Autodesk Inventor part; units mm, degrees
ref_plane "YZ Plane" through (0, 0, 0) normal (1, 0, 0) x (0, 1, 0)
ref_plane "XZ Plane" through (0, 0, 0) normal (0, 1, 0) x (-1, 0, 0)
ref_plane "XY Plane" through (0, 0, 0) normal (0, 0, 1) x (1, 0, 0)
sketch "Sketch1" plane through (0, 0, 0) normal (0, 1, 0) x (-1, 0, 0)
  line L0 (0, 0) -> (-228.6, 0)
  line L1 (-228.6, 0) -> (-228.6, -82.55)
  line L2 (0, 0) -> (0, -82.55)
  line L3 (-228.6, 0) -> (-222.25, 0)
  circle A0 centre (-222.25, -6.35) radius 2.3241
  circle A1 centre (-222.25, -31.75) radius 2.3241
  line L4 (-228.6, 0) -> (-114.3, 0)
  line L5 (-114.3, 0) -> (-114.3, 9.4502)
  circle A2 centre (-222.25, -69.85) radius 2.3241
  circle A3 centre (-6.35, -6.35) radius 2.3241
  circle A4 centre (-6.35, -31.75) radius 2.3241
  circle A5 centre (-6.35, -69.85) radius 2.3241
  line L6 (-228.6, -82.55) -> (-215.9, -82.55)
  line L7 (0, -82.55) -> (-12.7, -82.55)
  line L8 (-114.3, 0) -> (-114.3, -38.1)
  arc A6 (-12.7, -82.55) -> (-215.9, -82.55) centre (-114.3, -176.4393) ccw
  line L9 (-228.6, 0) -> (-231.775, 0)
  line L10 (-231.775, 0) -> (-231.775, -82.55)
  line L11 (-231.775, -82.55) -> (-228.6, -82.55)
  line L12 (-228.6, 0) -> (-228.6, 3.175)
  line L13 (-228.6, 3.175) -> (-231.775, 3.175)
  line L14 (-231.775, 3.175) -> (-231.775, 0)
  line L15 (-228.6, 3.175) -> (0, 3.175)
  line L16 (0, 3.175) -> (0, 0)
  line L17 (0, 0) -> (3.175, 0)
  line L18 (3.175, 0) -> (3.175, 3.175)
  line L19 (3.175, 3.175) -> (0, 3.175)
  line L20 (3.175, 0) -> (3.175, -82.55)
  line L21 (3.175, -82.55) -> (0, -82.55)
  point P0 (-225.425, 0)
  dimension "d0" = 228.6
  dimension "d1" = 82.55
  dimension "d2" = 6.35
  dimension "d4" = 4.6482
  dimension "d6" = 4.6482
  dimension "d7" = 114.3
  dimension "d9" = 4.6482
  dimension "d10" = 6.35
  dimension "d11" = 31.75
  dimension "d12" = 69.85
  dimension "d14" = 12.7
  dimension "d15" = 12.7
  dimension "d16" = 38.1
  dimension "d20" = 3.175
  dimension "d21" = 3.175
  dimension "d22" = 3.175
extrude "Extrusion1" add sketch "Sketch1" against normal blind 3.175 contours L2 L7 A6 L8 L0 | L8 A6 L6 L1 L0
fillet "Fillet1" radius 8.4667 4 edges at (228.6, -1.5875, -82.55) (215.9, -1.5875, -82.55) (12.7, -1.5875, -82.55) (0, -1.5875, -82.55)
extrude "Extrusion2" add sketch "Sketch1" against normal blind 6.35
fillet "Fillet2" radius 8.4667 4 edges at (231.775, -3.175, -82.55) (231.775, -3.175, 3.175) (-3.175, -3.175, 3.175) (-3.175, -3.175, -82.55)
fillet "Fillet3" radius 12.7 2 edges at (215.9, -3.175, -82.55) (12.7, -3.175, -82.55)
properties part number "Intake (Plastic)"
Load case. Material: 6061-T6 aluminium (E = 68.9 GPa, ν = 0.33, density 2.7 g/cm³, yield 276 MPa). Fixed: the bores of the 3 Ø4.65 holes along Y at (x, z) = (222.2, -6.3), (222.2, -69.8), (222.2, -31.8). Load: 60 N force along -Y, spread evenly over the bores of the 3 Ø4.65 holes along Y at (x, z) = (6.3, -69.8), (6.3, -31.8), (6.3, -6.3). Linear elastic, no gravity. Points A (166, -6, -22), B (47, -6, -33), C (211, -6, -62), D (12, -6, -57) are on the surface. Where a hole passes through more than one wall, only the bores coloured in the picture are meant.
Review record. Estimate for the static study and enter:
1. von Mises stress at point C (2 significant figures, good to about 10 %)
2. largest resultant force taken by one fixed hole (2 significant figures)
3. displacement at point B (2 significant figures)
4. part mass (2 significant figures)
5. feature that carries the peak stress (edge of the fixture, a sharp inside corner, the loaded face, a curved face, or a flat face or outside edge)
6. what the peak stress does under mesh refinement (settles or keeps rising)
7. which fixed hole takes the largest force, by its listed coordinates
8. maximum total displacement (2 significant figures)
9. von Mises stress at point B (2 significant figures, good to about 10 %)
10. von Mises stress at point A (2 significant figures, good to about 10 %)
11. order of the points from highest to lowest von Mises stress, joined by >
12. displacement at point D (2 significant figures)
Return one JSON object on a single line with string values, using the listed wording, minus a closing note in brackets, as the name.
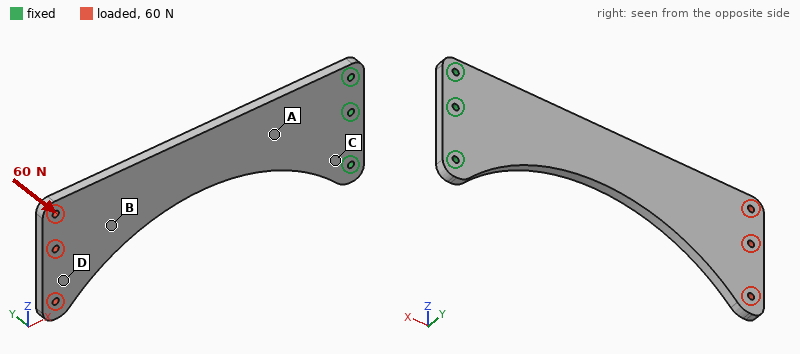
{"von Mises stress at point C": "18 MPa", "largest resultant force taken by one fixed hole": "110 N", "displacement at point B": "1.8 mm", "part mass": "240 g", "feature that carries the peak stress": "edge of the fixture", "what the peak stress does under mesh refinement": "keeps rising", "which fixed hole takes the largest force, by its listed coordinates": "(222.2, -31.8)", "maximum total displacement": "2.8 mm", "von Mises stress at point B": "6.4 MPa", "von Mises stress at point A": "27 MPa", "order of the points from highest to lowest von Mises stress, joined by >": "A > C > B > D", "displacement at point D": "2.5 mm"}
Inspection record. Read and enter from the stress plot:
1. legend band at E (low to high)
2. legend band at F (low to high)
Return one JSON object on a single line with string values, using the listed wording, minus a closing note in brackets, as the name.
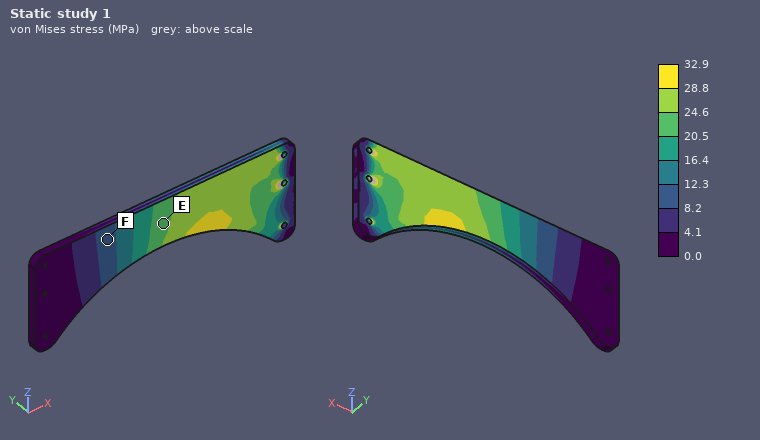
{"legend band at E": "20.5 to 24.6 MPa", "legend band at F": "8.2 to 12.3 MPa"}
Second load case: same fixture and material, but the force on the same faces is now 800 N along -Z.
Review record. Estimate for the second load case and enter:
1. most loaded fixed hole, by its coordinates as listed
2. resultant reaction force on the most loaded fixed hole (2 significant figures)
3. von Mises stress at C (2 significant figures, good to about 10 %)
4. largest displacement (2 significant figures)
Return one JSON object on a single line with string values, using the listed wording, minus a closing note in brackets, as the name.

{"most loaded fixed hole, by its coordinates as listed": "(222.2, -6.3)", "resultant reaction force on the most loaded fixed hole": "3.0 kN", "von Mises stress at C": "22 MPa", "largest displacement": "0.64 mm"}
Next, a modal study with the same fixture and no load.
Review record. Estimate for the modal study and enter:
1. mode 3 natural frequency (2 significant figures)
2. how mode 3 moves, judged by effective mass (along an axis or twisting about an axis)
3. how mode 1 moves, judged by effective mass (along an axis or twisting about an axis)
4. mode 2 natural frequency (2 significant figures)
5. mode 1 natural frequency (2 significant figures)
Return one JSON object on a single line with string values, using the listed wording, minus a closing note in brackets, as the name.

{"mode 3 natural frequency": "730 Hz", "how mode 3 moves, judged by effective mass": "along Z", "how mode 1 moves, judged by effective mass": "along Y", "mode 2 natural frequency": "520 Hz", "mode 1 natural frequency": "94 Hz"}
